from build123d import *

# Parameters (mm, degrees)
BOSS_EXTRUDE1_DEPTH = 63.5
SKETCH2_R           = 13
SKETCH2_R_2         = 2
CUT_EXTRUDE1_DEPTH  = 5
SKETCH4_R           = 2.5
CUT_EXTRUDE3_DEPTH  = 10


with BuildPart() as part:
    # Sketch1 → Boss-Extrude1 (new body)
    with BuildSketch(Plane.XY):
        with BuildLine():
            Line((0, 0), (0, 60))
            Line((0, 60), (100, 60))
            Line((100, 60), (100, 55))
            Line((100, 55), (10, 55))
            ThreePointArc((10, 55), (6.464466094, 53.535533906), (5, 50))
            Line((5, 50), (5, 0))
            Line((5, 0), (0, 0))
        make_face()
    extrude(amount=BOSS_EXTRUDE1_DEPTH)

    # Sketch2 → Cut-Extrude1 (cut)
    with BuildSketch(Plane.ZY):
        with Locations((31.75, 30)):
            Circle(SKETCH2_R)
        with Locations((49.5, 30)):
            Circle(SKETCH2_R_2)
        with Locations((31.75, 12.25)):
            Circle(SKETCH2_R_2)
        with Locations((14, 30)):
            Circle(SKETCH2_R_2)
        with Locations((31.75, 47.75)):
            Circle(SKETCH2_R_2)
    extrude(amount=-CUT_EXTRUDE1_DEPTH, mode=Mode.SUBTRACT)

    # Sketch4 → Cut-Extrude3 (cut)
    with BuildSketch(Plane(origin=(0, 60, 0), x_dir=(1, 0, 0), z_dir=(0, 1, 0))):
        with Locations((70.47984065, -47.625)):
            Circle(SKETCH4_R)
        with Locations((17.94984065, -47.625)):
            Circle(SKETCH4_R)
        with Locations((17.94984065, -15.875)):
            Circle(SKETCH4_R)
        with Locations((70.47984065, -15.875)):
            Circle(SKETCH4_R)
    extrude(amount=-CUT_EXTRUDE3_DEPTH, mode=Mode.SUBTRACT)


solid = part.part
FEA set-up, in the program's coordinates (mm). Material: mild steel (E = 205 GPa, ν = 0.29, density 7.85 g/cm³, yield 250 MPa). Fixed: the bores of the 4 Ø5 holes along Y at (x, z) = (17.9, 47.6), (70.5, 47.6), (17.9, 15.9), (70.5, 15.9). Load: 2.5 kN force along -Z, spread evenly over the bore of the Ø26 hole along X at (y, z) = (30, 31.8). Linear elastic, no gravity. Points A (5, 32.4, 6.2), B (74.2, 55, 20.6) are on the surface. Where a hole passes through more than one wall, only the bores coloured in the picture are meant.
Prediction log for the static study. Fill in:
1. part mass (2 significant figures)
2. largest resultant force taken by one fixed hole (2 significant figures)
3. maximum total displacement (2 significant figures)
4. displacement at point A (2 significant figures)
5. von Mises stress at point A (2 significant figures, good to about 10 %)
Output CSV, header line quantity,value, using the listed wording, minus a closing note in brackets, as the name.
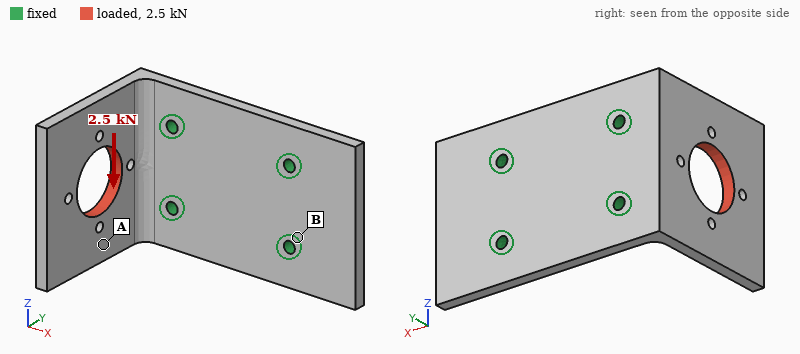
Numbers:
quantity,value
part mass,360 g
largest resultant force taken by one fixed hole,2.4 kN
maximum total displacement,97 µm
displacement at point A,53 µm
von Mises stress at point A,36 MPa
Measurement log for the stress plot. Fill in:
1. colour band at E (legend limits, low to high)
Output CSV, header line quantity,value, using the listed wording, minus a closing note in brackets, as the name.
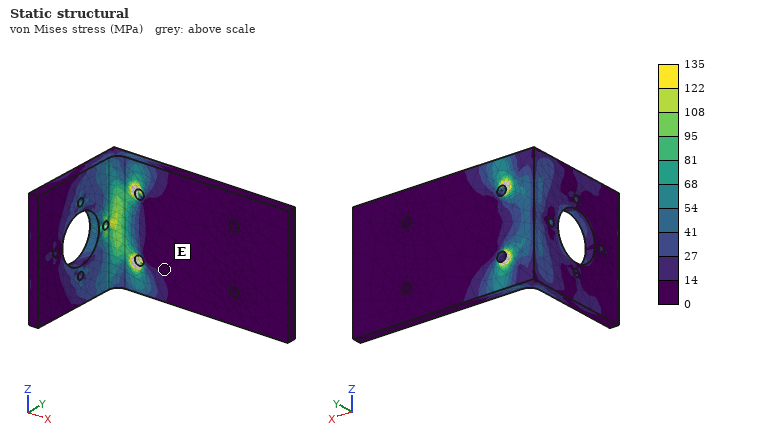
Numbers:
quantity,value
colour band at E,0 to 14 MPa
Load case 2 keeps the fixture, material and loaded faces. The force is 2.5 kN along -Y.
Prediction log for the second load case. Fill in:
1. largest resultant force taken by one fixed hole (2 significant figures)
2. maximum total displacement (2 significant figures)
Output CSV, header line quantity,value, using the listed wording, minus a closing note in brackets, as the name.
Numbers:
quantity,value
largest resultant force taken by one fixed hole,1.3 kN
maximum total displacement,0.14 mm
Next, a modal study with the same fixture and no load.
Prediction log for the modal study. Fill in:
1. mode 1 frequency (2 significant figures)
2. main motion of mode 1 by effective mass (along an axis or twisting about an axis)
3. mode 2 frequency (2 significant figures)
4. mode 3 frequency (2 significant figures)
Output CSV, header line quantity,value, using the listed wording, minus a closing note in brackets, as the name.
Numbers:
quantity,value
mode 1 frequency,930 Hz
main motion of mode 1 by effective mass,along X
mode 2 frequency,2100 Hz
mode 3 frequency,3100 Hz
